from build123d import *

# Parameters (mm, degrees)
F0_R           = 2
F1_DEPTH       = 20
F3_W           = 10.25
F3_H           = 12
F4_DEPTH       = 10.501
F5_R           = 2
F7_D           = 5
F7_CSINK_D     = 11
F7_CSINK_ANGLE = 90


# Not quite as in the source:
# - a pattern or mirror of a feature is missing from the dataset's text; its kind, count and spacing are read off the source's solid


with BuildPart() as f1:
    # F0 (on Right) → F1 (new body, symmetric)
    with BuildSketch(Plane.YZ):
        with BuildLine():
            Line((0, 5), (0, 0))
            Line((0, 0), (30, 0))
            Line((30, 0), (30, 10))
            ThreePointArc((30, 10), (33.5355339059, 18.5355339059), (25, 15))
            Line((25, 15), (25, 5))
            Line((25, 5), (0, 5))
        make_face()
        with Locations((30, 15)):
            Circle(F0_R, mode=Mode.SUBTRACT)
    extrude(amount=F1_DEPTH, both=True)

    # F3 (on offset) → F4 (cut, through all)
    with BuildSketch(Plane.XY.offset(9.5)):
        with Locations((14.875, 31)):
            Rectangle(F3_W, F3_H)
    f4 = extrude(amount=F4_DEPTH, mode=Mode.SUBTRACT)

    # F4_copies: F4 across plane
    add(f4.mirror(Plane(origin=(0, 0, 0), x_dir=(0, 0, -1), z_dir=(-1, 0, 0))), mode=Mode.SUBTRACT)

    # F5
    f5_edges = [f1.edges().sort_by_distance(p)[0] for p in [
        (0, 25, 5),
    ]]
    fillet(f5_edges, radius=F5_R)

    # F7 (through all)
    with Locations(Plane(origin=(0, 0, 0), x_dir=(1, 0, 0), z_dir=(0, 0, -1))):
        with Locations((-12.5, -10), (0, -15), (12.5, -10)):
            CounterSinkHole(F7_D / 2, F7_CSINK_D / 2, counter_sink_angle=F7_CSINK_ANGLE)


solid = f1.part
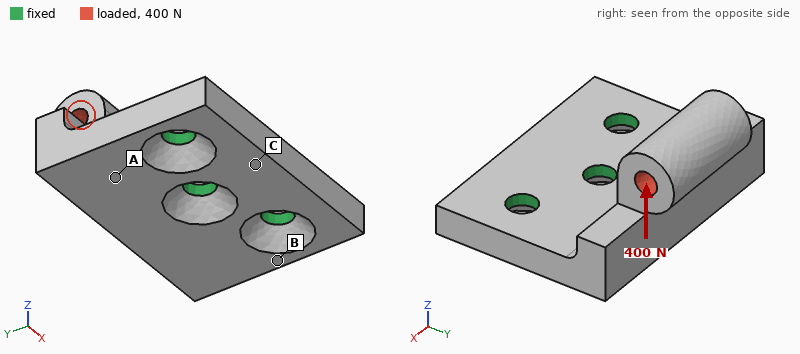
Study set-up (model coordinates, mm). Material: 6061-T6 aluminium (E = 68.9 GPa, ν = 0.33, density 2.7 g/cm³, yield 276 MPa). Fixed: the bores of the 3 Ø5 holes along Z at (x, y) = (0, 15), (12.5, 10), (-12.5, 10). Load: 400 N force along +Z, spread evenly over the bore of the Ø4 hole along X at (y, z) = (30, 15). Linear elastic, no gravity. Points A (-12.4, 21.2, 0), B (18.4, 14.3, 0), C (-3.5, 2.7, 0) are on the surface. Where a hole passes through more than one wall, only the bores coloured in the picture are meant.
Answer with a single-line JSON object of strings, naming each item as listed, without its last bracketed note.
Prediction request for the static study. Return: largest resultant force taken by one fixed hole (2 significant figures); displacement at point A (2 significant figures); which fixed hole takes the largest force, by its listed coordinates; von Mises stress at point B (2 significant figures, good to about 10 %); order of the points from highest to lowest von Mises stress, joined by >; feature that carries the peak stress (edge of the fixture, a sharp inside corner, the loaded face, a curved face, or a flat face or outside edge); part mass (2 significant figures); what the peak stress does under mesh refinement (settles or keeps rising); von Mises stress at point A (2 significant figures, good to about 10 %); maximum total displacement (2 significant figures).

{"largest resultant force taken by one fixed hole": "600 N", "displacement at point A": "17 µm", "which fixed hole takes the largest force, by its listed coordinates": "(0, 15)", "von Mises stress at point B": "28 MPa", "order of the points from highest to lowest von Mises stress, joined by >": "B > A > C", "feature that carries the peak stress": "edge of the fixture", "part mass": "21 g", "what the peak stress does under mesh refinement": "keeps rising", "von Mises stress at point A": "19 MPa", "maximum total displacement": "72 µm"}
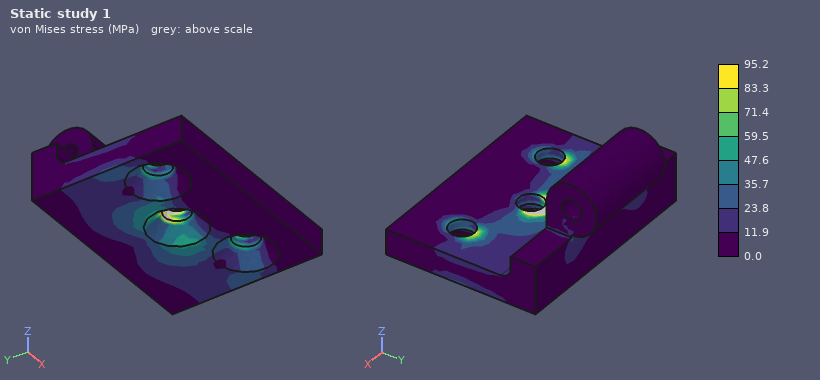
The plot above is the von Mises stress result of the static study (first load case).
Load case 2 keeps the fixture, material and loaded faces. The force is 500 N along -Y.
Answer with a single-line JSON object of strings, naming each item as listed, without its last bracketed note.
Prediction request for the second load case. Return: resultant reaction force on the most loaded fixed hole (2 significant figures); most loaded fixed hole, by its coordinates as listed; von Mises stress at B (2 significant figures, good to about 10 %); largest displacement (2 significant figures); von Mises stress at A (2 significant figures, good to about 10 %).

{"resultant reaction force on the most loaded fixed hole": "550 N", "most loaded fixed hole, by its coordinates as listed": "(0, 15)", "von Mises stress at B": "30 MPa", "largest displacement": "0.10 mm", "von Mises stress at A": "30 MPa"}
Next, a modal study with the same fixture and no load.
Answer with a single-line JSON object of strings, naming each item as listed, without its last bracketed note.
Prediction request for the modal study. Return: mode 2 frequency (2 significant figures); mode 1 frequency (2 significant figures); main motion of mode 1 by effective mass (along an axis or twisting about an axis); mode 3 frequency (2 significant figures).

{"mode 2 frequency": "8000 Hz", "mode 1 frequency": "4700 Hz", "main motion of mode 1 by effective mass": "along Z", "mode 3 frequency": "14 kHz"}
